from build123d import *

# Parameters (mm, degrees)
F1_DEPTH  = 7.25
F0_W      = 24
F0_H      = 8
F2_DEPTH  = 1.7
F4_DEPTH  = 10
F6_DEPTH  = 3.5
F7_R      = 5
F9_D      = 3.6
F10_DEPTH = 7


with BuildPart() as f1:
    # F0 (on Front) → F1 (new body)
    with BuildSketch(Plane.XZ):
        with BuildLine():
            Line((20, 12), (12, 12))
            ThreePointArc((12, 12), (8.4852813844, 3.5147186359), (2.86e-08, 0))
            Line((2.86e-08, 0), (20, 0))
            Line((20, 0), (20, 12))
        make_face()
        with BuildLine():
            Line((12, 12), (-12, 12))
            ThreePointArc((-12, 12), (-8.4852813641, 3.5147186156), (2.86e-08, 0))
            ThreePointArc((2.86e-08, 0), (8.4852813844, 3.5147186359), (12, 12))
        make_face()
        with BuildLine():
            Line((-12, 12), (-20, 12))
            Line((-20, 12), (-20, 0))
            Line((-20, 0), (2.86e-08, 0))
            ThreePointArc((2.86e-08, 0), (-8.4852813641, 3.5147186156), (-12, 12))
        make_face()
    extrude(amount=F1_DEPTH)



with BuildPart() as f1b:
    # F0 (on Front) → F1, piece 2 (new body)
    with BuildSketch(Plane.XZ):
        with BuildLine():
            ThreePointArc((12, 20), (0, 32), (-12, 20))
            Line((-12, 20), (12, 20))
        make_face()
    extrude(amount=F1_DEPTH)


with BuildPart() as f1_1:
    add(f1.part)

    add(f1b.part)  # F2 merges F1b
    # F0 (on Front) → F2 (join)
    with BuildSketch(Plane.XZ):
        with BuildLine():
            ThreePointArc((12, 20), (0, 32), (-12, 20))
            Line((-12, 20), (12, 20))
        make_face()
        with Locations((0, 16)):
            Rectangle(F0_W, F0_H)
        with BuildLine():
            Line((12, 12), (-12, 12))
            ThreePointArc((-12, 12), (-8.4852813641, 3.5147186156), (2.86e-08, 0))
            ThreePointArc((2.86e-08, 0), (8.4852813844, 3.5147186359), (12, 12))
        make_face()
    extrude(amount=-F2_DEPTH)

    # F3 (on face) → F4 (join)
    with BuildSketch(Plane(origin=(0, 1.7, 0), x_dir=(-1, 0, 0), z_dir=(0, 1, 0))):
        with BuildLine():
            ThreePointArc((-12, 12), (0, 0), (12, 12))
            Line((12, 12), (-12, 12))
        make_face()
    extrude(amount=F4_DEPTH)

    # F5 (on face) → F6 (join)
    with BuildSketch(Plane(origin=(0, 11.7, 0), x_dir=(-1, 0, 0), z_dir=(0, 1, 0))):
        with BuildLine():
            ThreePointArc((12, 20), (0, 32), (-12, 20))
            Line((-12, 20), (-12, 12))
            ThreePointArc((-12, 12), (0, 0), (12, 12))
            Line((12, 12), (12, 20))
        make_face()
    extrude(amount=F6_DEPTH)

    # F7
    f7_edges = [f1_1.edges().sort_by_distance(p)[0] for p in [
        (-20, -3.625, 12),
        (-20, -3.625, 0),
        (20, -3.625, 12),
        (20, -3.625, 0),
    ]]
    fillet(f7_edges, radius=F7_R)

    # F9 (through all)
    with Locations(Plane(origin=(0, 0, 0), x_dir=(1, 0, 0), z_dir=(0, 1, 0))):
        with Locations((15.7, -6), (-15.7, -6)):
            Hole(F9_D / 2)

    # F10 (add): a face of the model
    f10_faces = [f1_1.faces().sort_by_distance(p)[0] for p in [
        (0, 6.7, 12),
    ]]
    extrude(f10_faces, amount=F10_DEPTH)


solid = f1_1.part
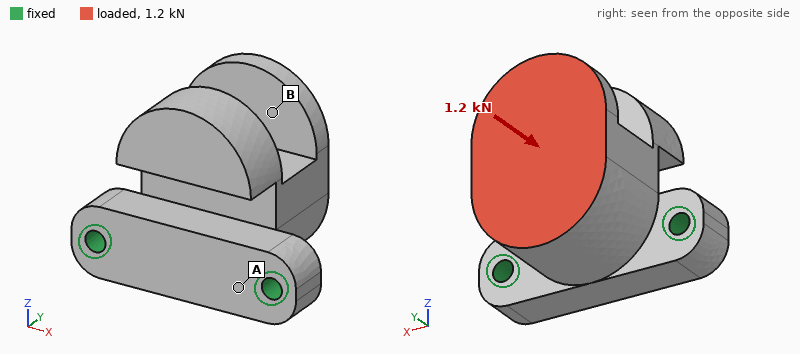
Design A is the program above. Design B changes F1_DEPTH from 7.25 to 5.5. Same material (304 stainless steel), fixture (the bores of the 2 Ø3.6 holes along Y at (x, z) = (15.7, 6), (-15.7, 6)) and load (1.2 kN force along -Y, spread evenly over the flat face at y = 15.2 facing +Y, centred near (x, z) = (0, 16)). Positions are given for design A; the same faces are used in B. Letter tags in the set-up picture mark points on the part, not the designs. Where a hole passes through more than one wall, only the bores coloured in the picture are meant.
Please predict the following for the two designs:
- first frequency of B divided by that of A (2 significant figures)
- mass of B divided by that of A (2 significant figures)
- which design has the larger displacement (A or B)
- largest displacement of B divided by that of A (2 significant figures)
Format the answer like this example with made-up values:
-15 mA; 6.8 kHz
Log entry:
0.98; 0.90; B; 1.3
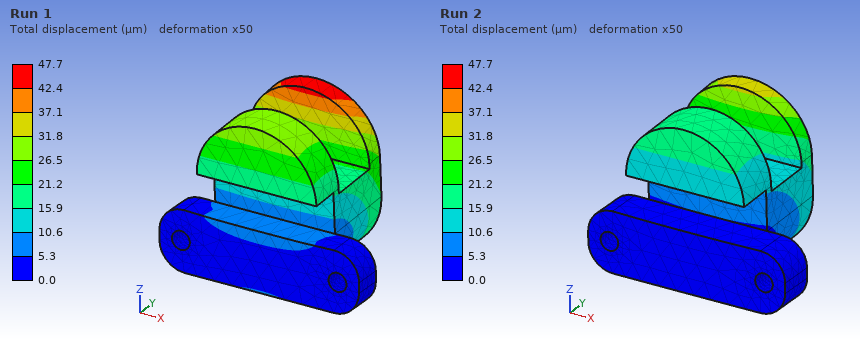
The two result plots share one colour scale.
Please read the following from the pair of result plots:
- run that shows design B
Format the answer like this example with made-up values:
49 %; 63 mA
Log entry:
Run 1
